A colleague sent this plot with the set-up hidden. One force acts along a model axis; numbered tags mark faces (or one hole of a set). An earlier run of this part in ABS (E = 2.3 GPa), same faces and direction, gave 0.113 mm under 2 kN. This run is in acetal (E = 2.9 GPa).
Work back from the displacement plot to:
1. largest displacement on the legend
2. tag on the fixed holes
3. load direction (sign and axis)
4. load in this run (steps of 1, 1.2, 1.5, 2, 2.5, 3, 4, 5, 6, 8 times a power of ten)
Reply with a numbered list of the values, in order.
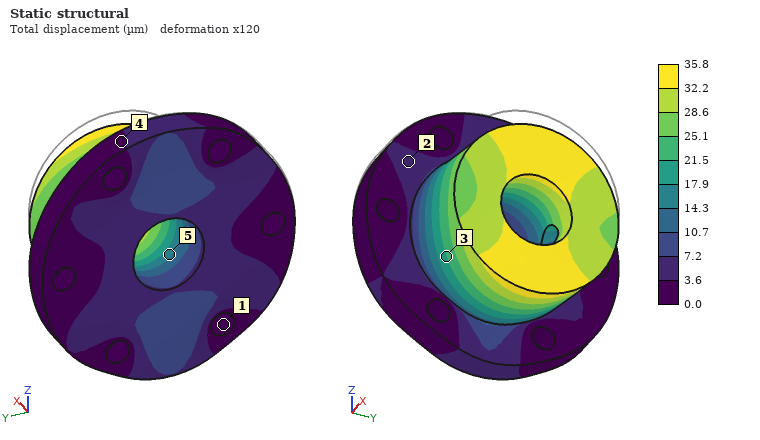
1. 35.8 µm
2. 1
3. -Z
4. 800 N
